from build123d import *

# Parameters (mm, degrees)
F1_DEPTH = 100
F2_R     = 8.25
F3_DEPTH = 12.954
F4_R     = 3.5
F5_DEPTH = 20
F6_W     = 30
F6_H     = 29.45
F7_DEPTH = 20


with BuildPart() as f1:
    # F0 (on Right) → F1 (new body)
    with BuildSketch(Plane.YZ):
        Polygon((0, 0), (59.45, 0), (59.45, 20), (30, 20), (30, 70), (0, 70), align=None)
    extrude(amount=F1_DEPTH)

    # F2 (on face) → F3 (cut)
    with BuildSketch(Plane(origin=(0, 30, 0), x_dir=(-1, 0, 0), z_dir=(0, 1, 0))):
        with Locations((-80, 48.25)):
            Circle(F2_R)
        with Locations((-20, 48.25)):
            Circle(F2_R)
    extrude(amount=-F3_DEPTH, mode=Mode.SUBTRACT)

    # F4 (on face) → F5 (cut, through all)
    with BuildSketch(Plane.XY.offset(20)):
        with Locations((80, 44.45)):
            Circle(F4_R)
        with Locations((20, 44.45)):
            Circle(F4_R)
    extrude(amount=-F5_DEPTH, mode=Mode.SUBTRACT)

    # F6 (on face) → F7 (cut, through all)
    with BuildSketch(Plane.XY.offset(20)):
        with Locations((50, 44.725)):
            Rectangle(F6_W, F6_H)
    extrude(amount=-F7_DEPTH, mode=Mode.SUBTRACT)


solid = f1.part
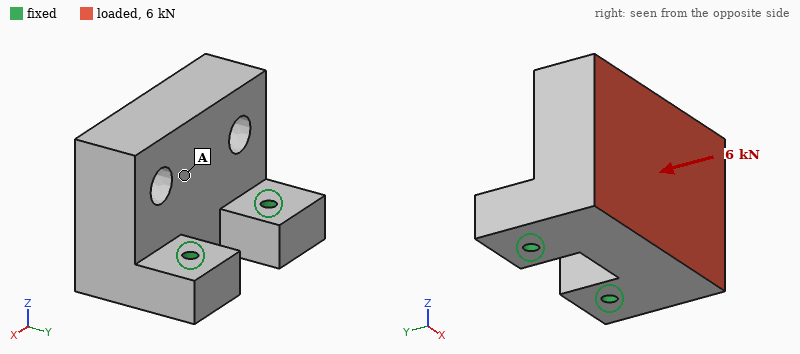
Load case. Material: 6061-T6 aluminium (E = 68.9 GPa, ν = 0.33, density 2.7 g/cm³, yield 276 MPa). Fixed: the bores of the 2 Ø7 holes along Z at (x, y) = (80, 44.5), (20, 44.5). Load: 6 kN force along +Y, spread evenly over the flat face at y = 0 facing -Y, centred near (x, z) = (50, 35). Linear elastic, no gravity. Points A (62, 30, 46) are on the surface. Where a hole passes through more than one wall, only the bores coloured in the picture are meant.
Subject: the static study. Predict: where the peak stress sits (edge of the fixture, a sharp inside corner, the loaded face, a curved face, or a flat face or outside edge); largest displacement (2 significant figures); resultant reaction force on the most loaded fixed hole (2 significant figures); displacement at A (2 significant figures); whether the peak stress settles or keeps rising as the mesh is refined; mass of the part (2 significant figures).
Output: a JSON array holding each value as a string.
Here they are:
["edge of the fixture", "93 µm", "3.0 kN", "48 µm", "keeps rising", "660 g"]
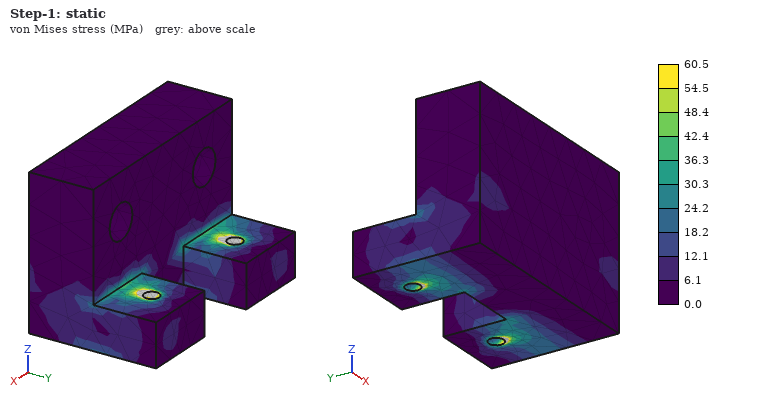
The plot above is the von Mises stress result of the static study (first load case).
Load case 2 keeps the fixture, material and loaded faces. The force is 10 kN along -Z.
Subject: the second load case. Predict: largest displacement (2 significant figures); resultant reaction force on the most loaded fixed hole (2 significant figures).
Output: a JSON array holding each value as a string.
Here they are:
["0.21 mm", "5.0 kN"]
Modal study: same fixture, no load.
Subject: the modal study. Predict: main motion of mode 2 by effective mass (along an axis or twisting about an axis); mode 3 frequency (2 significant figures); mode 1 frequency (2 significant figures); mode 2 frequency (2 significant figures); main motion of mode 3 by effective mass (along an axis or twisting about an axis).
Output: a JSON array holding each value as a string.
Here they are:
["along X", "5600 Hz", "1900 Hz", "3800 Hz", "along X"]
